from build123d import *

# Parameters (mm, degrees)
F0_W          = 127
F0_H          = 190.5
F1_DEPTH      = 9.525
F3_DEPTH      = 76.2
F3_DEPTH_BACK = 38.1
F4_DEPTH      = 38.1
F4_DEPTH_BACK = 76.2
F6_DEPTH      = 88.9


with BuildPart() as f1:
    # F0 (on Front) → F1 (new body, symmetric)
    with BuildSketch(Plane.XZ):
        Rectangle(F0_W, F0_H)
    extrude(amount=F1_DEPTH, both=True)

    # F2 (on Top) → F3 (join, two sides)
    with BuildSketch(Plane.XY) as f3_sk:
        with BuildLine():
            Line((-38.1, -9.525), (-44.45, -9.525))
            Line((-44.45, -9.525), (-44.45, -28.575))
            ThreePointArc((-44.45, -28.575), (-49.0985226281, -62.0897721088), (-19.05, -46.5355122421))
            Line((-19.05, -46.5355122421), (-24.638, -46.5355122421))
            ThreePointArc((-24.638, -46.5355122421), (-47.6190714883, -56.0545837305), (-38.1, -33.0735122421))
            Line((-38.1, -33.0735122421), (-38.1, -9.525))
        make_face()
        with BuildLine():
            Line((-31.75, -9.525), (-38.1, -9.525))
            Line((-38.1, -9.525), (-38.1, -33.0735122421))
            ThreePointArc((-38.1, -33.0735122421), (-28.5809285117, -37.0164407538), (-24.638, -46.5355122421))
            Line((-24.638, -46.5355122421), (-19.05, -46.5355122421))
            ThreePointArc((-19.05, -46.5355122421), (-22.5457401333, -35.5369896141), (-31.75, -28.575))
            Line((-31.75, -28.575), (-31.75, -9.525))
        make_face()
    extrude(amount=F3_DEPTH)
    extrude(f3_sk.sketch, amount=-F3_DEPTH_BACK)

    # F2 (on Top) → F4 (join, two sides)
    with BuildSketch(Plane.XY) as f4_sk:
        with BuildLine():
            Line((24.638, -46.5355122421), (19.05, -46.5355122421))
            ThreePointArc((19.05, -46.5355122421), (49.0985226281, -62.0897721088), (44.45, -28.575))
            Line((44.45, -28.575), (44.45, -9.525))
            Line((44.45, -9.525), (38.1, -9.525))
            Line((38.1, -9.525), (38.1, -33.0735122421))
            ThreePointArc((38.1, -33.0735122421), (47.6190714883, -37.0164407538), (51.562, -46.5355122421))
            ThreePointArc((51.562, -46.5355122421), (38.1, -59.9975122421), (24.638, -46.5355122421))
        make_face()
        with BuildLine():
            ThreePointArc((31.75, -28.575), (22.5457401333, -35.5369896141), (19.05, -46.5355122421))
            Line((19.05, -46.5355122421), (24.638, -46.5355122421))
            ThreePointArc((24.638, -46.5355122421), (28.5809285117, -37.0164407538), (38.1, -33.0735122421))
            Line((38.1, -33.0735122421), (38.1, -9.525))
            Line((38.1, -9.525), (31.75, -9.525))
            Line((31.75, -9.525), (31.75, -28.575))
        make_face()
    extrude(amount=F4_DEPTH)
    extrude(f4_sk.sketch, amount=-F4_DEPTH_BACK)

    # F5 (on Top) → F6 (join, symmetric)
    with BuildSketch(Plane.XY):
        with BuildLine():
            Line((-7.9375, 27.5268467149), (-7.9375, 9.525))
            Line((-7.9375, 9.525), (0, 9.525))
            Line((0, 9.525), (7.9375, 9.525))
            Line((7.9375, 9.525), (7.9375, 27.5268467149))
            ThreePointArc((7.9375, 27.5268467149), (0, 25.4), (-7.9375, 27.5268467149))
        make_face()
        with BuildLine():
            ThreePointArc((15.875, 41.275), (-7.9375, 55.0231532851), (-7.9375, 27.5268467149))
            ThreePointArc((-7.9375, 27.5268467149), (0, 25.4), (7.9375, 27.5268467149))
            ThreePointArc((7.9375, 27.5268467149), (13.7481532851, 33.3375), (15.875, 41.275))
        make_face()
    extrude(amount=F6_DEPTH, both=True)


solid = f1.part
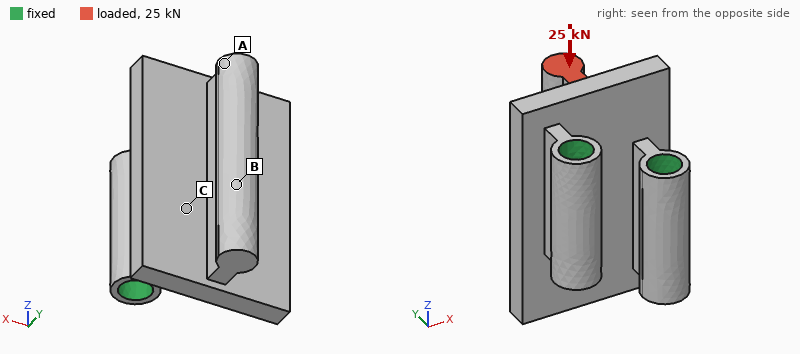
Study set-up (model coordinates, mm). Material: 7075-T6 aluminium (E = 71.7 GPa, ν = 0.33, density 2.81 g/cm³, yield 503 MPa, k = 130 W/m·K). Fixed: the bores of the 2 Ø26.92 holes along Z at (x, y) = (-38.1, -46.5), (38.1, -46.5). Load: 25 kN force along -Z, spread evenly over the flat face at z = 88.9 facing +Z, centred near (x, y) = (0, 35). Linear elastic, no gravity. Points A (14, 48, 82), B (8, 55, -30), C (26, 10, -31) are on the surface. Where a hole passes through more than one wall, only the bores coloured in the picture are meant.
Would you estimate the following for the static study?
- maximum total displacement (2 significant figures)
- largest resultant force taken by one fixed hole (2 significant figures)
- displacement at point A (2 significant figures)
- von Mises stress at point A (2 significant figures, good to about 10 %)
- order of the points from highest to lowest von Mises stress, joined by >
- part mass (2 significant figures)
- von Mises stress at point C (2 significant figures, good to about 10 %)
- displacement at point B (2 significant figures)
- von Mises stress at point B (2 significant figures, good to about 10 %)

0.11 mm
13 kN
0.099 mm
24 MPa
A > C > B
2.3 kg
16 MPa
0.056 mm
3.9 MPa
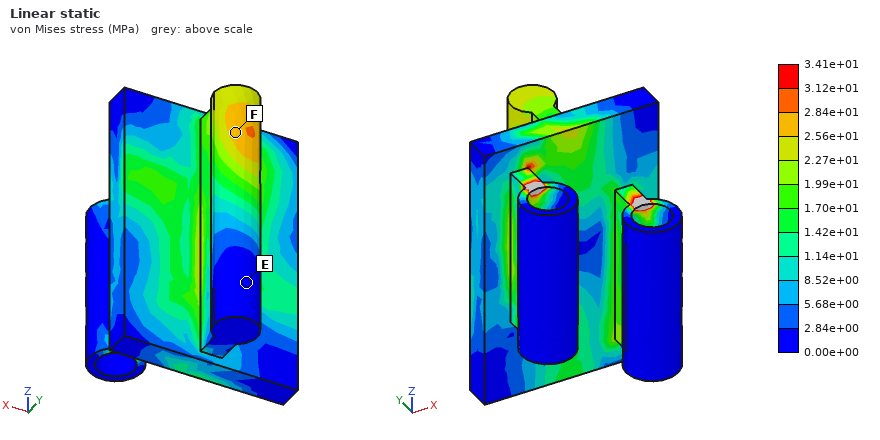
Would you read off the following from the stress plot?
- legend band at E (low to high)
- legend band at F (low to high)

0.00e+00 to 2.84e+00 MPa
2.56e+01 to 2.84e+01 MPa
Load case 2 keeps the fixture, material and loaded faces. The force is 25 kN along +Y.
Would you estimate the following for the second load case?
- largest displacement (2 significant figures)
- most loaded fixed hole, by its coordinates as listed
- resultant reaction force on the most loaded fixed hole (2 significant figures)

0.23 mm
(-38.1, -46.5)
15 kN
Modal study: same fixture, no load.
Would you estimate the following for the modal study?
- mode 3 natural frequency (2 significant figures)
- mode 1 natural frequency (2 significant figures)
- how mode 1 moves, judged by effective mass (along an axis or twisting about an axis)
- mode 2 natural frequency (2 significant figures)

3500 Hz
2500 Hz
along X
3500 Hz
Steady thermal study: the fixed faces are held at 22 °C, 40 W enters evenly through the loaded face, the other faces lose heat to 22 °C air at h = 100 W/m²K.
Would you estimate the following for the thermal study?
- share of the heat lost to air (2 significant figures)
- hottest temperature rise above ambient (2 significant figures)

51 %
15 K
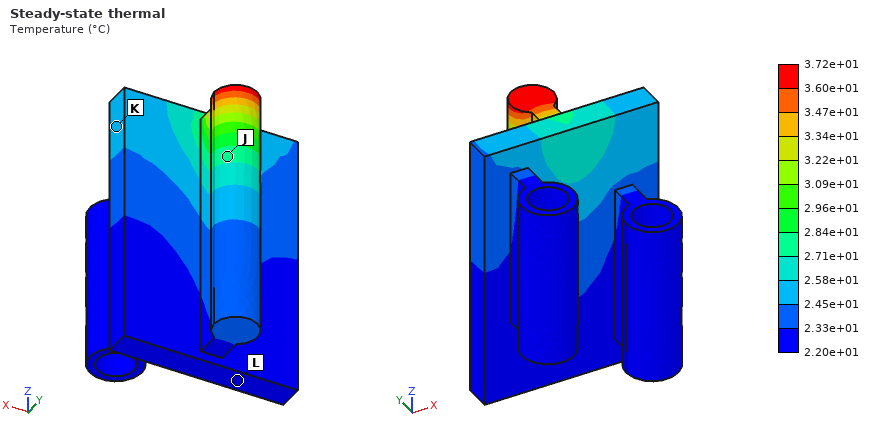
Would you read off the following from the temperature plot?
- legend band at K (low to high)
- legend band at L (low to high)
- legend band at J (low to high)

2.45e+01 to 2.58e+01 °C
2.20e+01 to 2.33e+01 °C
2.71e+01 to 2.84e+01 °C
